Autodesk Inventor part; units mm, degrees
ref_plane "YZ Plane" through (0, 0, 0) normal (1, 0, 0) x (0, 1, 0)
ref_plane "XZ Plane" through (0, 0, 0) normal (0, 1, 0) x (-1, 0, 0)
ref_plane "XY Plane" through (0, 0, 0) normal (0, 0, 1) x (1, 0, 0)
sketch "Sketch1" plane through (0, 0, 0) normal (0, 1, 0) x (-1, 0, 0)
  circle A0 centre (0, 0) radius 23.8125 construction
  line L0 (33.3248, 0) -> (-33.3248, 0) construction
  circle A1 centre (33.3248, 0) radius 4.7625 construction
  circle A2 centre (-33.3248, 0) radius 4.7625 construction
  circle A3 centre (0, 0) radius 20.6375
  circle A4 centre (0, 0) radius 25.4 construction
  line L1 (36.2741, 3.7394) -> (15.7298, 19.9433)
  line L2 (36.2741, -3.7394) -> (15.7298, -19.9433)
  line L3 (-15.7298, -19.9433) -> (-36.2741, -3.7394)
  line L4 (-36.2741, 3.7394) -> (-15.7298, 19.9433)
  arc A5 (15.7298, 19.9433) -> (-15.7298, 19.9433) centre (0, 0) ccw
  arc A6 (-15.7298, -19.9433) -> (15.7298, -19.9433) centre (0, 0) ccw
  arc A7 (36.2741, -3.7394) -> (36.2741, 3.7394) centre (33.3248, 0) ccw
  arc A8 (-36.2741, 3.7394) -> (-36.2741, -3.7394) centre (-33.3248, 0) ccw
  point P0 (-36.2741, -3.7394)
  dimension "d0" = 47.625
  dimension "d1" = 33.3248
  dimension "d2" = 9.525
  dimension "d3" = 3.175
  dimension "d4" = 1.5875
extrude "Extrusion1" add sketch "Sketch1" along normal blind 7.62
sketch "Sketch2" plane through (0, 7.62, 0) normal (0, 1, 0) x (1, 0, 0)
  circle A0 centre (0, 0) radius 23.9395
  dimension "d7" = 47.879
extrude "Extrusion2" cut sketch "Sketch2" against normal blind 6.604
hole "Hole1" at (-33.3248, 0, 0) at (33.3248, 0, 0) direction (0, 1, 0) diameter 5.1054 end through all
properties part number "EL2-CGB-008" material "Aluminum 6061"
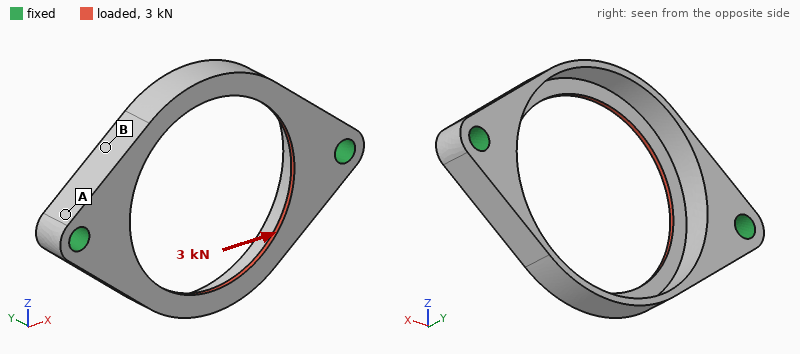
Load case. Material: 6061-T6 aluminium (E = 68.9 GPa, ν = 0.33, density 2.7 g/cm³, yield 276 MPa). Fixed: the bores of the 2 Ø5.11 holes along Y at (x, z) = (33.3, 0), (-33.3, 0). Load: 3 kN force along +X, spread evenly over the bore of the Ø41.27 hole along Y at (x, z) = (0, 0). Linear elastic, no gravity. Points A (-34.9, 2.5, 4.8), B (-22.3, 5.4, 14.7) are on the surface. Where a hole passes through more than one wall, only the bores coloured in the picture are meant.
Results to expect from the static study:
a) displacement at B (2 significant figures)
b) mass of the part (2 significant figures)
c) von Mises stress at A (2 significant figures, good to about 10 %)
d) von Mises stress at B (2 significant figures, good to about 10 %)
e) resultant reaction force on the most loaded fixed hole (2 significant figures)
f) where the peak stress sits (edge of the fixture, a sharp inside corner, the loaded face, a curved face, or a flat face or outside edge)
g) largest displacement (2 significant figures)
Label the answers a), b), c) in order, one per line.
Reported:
a) 21 µm
b) 14 g
c) 25 MPa
d) 57 MPa
e) 1.5 kN
f) the loaded face
g) 77 µm
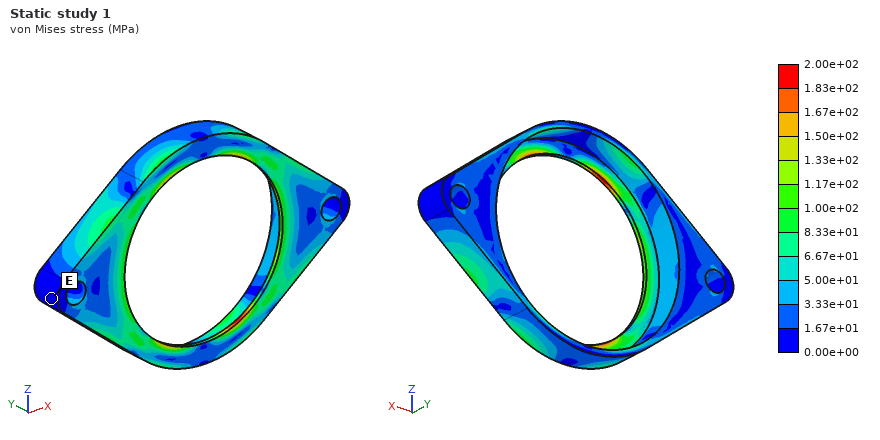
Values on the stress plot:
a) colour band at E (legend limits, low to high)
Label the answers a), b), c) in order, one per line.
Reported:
a) 0.00e+00 to 1.67e+01 MPa
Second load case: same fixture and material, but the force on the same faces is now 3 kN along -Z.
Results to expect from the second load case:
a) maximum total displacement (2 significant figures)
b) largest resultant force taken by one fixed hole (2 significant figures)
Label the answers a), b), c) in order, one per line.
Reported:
a) 0.11 mm
b) 1.5 kN
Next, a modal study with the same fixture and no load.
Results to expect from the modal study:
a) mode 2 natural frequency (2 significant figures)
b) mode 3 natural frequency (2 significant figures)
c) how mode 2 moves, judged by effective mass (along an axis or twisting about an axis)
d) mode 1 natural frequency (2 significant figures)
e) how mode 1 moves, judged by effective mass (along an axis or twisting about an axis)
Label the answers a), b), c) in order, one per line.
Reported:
a) 7700 Hz
b) 10 kHz
c) along Y
d) 7200 Hz
e) twisting about X
